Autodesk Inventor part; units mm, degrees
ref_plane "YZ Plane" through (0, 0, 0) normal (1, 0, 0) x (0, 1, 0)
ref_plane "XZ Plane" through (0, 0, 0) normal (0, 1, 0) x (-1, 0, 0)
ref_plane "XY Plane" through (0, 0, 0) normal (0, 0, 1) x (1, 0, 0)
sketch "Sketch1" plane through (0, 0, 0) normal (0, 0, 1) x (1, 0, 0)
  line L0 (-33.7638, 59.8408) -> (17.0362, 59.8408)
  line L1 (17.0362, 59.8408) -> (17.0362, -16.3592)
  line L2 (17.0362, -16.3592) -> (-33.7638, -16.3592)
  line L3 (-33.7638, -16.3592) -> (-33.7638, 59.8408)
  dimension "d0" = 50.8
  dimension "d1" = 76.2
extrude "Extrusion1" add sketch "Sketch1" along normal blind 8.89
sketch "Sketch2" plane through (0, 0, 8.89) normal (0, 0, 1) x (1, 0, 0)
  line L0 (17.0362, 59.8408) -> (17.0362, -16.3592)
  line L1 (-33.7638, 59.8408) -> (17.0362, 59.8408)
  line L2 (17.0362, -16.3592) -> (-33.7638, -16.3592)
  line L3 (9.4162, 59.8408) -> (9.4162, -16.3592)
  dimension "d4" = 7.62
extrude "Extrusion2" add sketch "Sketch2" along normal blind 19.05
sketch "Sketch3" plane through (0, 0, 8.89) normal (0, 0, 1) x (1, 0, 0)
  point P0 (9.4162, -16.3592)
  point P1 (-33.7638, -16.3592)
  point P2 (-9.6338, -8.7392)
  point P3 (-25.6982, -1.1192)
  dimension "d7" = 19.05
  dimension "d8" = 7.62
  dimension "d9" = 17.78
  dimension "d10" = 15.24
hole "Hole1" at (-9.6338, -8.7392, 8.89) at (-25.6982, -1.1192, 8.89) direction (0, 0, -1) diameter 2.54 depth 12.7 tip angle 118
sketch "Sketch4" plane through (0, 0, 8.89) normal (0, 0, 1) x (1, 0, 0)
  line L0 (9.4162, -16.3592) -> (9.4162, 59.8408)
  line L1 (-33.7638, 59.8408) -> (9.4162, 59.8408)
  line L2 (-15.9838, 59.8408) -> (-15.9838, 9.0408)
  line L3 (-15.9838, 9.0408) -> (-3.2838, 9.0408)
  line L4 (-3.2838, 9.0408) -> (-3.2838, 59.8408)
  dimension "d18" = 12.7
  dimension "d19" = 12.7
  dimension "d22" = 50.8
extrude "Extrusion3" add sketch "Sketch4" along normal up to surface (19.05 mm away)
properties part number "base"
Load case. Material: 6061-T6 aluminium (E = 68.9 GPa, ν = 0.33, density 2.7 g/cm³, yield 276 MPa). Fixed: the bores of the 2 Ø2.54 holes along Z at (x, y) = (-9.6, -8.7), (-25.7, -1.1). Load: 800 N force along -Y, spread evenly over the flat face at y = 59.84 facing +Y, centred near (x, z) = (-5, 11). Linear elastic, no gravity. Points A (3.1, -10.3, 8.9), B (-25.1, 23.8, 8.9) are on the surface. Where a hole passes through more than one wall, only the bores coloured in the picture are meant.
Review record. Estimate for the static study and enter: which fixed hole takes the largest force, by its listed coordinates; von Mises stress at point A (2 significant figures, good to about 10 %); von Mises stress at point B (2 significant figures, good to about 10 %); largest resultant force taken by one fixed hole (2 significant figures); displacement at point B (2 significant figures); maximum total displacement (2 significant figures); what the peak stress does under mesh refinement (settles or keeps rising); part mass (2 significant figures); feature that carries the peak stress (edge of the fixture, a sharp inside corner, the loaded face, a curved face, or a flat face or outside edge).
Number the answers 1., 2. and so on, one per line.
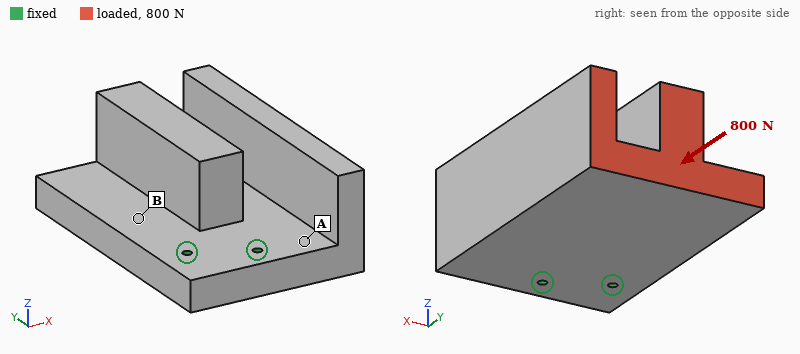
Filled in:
1. (-9.6, -8.7)
2. 7.4 MPa
3. 2.7 MPa
4. 910 N
5. 10 µm
6. 42 µm
7. keeps rising
8. 160 g
9. edge of the fixture
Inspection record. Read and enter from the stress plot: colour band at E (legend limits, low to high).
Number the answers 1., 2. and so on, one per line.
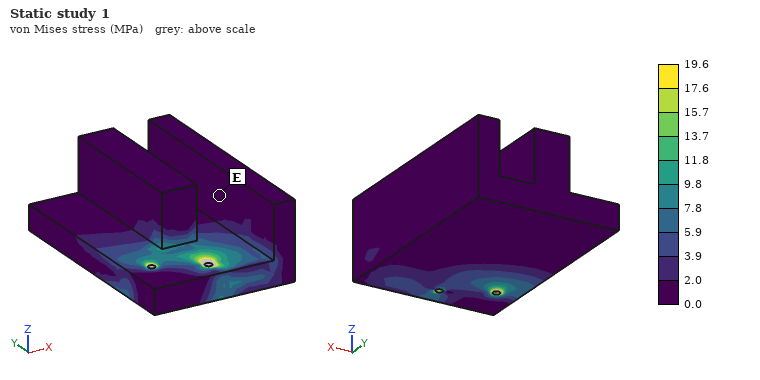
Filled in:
1. 0.0 to 2.0 MPa
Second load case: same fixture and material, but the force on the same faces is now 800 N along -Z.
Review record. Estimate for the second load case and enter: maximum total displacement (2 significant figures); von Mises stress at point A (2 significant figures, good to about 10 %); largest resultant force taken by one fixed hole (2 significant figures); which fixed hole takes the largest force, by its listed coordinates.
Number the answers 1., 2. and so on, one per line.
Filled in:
1. 0.40 mm
2. 54 MPa
3. 840 N
4. (-25.7, -1.1)
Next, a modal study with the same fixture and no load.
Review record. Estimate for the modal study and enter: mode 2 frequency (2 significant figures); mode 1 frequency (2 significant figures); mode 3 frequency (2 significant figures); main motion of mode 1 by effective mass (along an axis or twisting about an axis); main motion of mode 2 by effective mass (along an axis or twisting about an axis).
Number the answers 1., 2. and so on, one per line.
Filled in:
1. 2600 Hz
2. 1100 Hz
3. 3400 Hz
4. along Z
5. along X
